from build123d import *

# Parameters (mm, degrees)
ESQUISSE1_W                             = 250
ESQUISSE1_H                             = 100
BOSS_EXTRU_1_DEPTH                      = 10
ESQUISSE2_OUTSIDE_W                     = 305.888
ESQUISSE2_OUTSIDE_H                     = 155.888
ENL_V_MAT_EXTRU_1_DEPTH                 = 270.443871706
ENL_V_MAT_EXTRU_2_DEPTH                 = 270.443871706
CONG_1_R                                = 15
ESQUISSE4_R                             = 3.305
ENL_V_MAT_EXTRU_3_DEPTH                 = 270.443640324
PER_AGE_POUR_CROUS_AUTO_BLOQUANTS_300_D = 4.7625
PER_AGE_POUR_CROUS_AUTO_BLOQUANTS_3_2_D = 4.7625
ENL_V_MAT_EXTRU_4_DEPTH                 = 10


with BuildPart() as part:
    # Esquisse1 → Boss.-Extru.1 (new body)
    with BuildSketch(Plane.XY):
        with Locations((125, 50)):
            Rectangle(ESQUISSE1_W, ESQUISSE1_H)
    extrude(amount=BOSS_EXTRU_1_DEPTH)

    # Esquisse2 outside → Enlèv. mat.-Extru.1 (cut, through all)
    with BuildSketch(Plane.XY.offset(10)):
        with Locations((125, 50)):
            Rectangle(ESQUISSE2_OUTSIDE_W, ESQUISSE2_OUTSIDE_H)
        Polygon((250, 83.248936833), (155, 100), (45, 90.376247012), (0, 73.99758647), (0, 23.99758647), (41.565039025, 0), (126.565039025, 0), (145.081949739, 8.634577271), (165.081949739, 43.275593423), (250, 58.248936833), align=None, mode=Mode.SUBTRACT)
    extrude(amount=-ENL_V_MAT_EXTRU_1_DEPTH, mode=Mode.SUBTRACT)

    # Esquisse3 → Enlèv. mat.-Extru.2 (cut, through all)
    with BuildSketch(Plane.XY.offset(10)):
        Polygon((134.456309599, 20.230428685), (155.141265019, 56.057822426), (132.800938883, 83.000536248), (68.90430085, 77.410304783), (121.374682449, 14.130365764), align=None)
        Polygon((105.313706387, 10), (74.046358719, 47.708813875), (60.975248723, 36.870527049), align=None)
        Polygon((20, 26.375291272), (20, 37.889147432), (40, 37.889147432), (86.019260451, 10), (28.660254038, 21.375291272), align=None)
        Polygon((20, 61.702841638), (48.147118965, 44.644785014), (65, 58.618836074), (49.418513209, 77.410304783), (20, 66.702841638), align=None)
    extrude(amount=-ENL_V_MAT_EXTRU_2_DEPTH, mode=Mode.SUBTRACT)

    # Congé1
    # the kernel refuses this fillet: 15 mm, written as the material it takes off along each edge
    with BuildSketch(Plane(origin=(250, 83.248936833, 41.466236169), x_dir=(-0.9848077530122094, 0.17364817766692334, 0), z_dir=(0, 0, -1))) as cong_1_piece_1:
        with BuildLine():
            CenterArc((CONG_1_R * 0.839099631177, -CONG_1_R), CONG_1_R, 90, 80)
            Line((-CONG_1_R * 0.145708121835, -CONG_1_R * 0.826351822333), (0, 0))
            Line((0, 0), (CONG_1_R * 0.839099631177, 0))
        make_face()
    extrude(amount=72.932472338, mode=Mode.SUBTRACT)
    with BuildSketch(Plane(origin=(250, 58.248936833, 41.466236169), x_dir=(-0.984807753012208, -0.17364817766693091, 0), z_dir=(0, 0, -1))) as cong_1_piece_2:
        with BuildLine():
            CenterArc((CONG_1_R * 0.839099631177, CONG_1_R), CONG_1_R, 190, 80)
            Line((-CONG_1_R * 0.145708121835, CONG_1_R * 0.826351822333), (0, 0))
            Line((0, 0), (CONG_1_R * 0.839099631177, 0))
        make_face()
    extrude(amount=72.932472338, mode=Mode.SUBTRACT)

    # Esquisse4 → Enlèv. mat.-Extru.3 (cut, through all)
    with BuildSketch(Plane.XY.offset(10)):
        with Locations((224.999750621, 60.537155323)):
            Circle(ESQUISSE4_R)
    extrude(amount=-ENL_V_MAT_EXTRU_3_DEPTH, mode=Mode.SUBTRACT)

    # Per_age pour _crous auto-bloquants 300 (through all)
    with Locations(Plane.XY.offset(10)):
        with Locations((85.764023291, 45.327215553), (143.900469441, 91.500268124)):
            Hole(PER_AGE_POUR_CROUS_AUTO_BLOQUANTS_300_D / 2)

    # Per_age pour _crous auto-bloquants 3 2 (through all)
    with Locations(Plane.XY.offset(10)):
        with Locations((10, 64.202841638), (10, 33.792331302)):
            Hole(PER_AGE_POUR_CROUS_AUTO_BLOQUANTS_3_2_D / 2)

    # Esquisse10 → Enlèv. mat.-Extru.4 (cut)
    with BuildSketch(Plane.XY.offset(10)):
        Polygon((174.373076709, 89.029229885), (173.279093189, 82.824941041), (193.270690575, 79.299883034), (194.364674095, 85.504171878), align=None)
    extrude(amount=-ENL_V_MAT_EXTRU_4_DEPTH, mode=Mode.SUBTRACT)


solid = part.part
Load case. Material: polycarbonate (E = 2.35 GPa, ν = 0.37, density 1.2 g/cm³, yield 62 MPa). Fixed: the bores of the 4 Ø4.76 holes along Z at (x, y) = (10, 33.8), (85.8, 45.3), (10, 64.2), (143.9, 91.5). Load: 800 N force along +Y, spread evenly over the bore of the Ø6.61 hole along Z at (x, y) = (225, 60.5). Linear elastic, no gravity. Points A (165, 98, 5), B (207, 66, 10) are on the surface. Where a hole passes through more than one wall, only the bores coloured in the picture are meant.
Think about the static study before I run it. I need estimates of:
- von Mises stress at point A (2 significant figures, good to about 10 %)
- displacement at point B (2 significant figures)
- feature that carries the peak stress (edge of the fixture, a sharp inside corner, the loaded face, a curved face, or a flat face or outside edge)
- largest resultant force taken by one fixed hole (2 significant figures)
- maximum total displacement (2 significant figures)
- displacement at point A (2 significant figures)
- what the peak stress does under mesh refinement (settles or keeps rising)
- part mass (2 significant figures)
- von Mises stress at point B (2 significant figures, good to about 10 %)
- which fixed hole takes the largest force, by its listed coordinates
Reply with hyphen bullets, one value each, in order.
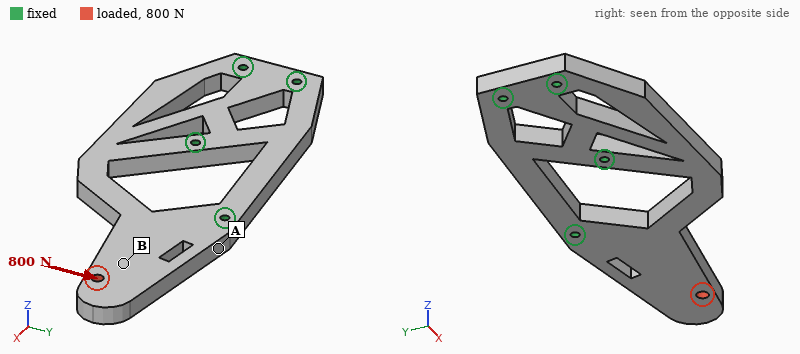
- 9.9 MPa
- 1.6 mm
- edge of the fixture
- 930 N
- 2.9 mm
- 0.49 mm
- keeps rising
- 140 g
- 4.2 MPa
- (143.9, 91.5)
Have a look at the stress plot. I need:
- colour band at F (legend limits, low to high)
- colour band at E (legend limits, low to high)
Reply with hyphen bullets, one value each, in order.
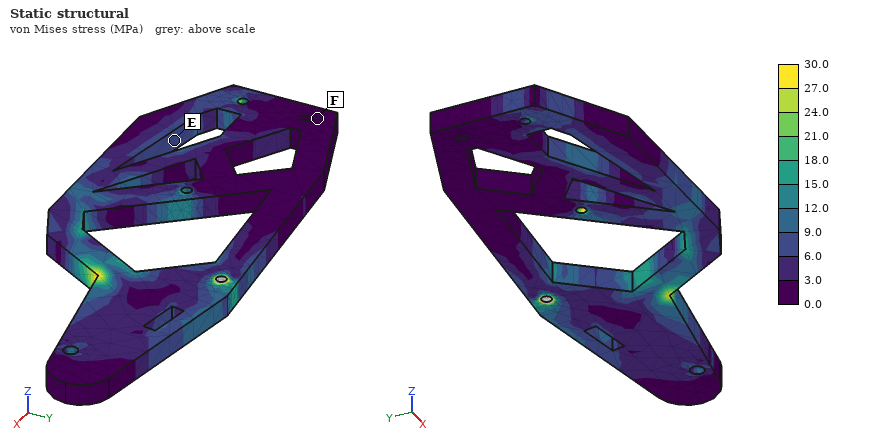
- 0.0 to 3.0 MPa
- 6.0 to 9.0 MPa
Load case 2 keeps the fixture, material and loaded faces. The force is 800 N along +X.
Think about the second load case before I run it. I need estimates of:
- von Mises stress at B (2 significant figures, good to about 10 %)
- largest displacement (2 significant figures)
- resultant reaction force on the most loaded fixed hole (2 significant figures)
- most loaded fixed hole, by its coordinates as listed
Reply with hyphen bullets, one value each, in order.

- 2.7 MPa
- 0.99 mm
- 500 N
- (143.9, 91.5)
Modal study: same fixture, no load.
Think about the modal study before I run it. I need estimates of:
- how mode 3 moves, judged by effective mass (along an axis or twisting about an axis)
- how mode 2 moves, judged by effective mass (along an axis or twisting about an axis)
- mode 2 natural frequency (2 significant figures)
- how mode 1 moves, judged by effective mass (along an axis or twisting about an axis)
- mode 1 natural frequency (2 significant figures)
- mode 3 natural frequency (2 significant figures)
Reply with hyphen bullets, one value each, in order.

- along Y
- along Z
- 460 Hz
- along Z
- 200 Hz
- 590 Hz
